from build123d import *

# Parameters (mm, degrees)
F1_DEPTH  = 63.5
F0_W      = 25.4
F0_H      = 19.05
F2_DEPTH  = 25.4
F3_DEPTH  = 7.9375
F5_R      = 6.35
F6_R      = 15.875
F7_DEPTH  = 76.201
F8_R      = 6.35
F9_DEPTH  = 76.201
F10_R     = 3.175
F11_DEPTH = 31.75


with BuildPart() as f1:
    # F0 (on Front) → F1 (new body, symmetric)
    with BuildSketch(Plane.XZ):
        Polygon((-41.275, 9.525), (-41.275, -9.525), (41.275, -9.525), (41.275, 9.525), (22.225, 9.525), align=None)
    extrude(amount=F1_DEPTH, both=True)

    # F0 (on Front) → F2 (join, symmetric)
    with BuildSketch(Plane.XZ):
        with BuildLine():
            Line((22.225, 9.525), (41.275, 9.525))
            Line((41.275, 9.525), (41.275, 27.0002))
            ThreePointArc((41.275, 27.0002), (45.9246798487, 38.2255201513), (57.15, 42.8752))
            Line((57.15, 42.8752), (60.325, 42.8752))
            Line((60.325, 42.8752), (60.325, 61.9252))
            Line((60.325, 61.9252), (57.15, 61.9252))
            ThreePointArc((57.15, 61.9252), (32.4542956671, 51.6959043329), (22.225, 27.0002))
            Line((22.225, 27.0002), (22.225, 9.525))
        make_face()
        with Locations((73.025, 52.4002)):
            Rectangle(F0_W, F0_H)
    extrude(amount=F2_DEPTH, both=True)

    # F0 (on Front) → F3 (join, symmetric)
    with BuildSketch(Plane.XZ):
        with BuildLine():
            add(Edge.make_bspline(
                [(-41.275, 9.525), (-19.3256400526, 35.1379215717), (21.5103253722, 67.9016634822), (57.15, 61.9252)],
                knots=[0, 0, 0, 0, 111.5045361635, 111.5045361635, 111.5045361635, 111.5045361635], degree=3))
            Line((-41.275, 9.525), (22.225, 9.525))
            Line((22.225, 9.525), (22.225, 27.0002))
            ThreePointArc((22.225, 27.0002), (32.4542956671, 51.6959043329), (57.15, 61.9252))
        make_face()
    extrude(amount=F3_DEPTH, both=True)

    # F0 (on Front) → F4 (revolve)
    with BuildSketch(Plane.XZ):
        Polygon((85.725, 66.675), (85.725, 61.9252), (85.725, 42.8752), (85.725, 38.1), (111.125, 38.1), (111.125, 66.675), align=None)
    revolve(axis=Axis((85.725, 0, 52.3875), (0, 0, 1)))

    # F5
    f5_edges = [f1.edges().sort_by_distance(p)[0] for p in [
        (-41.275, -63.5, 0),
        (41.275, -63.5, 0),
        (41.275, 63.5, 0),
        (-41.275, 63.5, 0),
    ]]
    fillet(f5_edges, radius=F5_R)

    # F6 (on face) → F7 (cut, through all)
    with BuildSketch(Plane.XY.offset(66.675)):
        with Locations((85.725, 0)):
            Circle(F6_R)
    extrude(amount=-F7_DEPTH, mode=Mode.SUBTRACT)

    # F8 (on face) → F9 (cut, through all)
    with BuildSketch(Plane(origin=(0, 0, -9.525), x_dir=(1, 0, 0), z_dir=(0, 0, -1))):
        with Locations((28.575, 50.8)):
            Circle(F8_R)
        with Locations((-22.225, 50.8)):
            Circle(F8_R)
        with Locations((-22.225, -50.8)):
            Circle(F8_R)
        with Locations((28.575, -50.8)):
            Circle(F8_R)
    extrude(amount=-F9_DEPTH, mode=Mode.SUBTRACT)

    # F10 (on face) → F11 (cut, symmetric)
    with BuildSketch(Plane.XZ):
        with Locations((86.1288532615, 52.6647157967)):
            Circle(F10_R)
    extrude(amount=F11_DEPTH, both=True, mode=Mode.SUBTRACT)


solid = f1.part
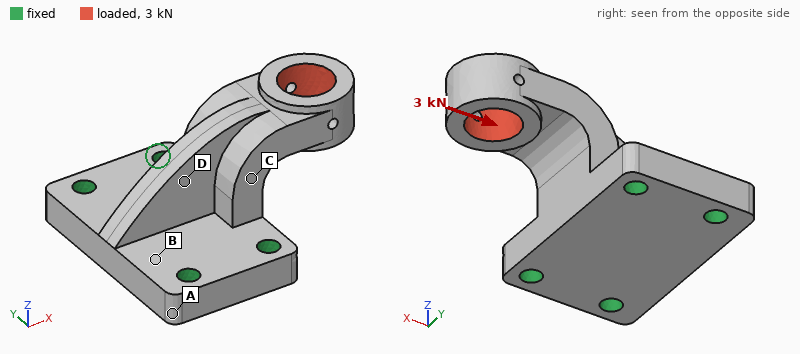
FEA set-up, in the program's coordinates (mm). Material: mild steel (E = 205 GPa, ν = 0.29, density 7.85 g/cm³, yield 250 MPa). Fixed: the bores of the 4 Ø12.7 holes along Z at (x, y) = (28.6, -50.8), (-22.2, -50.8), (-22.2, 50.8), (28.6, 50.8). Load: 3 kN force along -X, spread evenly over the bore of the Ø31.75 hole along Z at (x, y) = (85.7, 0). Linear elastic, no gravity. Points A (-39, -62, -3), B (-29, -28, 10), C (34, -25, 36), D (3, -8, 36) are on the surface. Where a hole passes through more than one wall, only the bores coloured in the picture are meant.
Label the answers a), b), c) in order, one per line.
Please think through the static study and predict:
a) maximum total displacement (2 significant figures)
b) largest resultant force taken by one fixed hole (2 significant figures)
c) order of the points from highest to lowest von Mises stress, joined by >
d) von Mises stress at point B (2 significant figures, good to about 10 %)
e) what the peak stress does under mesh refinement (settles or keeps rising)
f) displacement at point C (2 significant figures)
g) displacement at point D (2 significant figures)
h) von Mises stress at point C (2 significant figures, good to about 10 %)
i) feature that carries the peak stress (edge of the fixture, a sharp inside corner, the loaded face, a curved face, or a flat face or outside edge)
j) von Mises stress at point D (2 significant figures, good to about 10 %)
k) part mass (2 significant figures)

a) 23 µm
b) 1.7 kN
c) D > B > C > A
d) 5.7 MPa
e) keeps rising
f) 6.2 µm
g) 5.1 µm
h) 2.7 MPa
i) edge of the fixture
j) 7.5 MPa
k) 2.5 kg
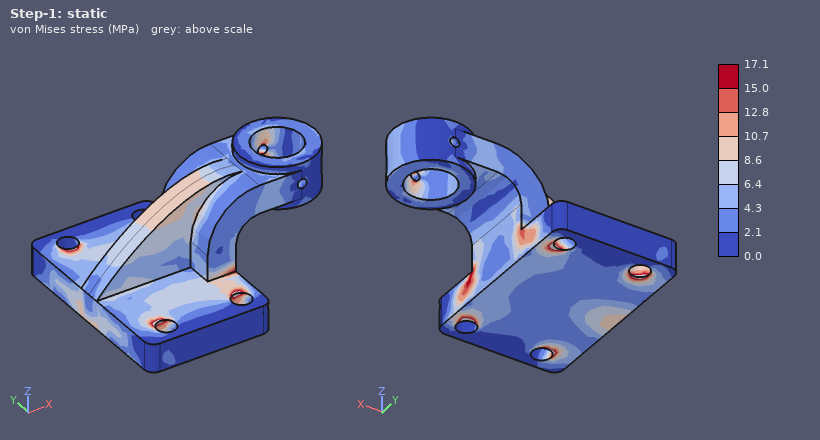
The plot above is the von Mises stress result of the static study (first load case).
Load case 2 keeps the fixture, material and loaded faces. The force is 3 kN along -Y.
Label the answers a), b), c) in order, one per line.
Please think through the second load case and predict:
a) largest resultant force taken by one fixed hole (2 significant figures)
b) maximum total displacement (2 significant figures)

a) 2.6 kN
b) 58 µm
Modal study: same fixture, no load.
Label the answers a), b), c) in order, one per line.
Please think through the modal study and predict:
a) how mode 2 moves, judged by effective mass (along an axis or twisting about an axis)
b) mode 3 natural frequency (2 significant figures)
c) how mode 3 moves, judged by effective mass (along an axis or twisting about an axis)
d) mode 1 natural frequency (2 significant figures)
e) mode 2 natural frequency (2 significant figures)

a) along Y
b) 4400 Hz
c) along X
d) 2000 Hz
e) 2300 Hz
